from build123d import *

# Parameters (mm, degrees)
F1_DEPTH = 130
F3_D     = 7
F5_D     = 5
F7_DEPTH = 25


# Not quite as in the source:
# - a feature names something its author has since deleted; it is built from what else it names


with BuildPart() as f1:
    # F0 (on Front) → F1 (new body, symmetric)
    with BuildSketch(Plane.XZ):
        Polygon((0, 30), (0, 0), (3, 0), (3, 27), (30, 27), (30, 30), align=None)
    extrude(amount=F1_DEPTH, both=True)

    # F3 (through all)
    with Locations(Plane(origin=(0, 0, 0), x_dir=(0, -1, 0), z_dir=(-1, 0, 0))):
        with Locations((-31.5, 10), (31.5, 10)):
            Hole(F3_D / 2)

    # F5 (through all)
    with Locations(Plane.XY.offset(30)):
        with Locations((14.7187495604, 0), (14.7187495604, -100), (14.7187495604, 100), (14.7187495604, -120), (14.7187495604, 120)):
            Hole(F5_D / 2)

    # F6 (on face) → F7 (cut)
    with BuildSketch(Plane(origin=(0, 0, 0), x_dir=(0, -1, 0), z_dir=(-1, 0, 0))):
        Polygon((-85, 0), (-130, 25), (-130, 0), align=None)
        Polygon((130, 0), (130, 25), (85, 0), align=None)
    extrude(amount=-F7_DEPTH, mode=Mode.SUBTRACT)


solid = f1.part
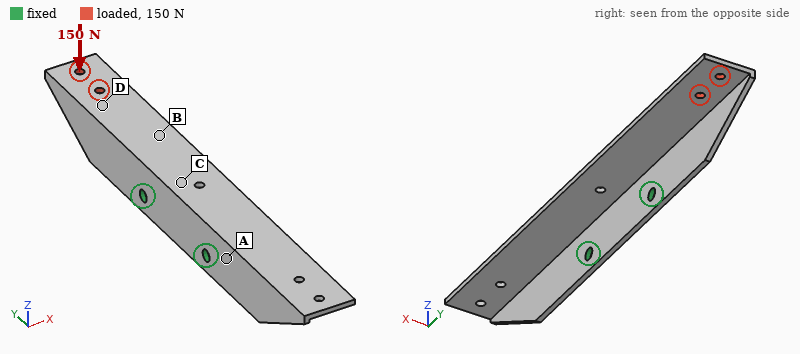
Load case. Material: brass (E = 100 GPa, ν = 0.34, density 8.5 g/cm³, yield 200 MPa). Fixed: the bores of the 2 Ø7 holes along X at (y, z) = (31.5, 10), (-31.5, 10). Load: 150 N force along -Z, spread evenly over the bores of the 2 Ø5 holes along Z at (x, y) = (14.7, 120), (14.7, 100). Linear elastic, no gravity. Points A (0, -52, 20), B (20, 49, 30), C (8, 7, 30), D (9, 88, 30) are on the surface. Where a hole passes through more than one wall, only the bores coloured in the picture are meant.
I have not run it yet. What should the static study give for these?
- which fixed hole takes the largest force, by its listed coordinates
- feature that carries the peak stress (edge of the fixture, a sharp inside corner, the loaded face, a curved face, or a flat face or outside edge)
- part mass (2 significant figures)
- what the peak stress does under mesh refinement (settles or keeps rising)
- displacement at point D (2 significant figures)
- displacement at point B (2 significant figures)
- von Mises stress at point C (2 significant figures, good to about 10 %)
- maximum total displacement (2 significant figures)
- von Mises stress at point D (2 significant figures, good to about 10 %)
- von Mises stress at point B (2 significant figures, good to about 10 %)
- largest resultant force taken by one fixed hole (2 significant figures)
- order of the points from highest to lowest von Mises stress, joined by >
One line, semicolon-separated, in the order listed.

(31.5, 10); edge of the fixture; 340 g; keeps rising; 0.099 mm; 0.073 mm; 8.9 MPa; 0.35 mm; 22 MPa; 15 MPa; 350 N; D > B > C > A
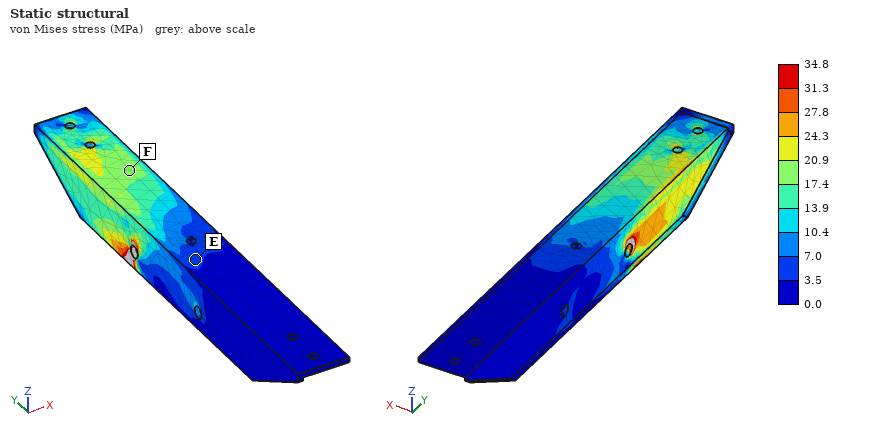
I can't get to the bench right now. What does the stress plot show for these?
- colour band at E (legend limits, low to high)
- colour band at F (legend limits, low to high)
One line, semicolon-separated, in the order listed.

3.5 to 7.0 MPa; 17.4 to 20.9 MPa
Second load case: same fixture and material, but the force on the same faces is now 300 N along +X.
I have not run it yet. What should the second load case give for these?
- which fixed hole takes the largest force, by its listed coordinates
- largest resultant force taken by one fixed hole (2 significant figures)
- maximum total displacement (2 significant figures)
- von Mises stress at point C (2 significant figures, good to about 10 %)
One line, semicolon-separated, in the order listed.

(31.5, 10); 640 N; 0.52 mm; 21 MPa
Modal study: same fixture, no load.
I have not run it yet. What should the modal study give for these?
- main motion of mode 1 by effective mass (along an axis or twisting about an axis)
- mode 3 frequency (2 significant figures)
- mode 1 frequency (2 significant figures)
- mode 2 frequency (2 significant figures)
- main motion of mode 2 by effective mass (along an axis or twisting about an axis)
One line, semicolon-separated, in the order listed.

twisting about Z; 710 Hz; 450 Hz; 580 Hz; along Z
